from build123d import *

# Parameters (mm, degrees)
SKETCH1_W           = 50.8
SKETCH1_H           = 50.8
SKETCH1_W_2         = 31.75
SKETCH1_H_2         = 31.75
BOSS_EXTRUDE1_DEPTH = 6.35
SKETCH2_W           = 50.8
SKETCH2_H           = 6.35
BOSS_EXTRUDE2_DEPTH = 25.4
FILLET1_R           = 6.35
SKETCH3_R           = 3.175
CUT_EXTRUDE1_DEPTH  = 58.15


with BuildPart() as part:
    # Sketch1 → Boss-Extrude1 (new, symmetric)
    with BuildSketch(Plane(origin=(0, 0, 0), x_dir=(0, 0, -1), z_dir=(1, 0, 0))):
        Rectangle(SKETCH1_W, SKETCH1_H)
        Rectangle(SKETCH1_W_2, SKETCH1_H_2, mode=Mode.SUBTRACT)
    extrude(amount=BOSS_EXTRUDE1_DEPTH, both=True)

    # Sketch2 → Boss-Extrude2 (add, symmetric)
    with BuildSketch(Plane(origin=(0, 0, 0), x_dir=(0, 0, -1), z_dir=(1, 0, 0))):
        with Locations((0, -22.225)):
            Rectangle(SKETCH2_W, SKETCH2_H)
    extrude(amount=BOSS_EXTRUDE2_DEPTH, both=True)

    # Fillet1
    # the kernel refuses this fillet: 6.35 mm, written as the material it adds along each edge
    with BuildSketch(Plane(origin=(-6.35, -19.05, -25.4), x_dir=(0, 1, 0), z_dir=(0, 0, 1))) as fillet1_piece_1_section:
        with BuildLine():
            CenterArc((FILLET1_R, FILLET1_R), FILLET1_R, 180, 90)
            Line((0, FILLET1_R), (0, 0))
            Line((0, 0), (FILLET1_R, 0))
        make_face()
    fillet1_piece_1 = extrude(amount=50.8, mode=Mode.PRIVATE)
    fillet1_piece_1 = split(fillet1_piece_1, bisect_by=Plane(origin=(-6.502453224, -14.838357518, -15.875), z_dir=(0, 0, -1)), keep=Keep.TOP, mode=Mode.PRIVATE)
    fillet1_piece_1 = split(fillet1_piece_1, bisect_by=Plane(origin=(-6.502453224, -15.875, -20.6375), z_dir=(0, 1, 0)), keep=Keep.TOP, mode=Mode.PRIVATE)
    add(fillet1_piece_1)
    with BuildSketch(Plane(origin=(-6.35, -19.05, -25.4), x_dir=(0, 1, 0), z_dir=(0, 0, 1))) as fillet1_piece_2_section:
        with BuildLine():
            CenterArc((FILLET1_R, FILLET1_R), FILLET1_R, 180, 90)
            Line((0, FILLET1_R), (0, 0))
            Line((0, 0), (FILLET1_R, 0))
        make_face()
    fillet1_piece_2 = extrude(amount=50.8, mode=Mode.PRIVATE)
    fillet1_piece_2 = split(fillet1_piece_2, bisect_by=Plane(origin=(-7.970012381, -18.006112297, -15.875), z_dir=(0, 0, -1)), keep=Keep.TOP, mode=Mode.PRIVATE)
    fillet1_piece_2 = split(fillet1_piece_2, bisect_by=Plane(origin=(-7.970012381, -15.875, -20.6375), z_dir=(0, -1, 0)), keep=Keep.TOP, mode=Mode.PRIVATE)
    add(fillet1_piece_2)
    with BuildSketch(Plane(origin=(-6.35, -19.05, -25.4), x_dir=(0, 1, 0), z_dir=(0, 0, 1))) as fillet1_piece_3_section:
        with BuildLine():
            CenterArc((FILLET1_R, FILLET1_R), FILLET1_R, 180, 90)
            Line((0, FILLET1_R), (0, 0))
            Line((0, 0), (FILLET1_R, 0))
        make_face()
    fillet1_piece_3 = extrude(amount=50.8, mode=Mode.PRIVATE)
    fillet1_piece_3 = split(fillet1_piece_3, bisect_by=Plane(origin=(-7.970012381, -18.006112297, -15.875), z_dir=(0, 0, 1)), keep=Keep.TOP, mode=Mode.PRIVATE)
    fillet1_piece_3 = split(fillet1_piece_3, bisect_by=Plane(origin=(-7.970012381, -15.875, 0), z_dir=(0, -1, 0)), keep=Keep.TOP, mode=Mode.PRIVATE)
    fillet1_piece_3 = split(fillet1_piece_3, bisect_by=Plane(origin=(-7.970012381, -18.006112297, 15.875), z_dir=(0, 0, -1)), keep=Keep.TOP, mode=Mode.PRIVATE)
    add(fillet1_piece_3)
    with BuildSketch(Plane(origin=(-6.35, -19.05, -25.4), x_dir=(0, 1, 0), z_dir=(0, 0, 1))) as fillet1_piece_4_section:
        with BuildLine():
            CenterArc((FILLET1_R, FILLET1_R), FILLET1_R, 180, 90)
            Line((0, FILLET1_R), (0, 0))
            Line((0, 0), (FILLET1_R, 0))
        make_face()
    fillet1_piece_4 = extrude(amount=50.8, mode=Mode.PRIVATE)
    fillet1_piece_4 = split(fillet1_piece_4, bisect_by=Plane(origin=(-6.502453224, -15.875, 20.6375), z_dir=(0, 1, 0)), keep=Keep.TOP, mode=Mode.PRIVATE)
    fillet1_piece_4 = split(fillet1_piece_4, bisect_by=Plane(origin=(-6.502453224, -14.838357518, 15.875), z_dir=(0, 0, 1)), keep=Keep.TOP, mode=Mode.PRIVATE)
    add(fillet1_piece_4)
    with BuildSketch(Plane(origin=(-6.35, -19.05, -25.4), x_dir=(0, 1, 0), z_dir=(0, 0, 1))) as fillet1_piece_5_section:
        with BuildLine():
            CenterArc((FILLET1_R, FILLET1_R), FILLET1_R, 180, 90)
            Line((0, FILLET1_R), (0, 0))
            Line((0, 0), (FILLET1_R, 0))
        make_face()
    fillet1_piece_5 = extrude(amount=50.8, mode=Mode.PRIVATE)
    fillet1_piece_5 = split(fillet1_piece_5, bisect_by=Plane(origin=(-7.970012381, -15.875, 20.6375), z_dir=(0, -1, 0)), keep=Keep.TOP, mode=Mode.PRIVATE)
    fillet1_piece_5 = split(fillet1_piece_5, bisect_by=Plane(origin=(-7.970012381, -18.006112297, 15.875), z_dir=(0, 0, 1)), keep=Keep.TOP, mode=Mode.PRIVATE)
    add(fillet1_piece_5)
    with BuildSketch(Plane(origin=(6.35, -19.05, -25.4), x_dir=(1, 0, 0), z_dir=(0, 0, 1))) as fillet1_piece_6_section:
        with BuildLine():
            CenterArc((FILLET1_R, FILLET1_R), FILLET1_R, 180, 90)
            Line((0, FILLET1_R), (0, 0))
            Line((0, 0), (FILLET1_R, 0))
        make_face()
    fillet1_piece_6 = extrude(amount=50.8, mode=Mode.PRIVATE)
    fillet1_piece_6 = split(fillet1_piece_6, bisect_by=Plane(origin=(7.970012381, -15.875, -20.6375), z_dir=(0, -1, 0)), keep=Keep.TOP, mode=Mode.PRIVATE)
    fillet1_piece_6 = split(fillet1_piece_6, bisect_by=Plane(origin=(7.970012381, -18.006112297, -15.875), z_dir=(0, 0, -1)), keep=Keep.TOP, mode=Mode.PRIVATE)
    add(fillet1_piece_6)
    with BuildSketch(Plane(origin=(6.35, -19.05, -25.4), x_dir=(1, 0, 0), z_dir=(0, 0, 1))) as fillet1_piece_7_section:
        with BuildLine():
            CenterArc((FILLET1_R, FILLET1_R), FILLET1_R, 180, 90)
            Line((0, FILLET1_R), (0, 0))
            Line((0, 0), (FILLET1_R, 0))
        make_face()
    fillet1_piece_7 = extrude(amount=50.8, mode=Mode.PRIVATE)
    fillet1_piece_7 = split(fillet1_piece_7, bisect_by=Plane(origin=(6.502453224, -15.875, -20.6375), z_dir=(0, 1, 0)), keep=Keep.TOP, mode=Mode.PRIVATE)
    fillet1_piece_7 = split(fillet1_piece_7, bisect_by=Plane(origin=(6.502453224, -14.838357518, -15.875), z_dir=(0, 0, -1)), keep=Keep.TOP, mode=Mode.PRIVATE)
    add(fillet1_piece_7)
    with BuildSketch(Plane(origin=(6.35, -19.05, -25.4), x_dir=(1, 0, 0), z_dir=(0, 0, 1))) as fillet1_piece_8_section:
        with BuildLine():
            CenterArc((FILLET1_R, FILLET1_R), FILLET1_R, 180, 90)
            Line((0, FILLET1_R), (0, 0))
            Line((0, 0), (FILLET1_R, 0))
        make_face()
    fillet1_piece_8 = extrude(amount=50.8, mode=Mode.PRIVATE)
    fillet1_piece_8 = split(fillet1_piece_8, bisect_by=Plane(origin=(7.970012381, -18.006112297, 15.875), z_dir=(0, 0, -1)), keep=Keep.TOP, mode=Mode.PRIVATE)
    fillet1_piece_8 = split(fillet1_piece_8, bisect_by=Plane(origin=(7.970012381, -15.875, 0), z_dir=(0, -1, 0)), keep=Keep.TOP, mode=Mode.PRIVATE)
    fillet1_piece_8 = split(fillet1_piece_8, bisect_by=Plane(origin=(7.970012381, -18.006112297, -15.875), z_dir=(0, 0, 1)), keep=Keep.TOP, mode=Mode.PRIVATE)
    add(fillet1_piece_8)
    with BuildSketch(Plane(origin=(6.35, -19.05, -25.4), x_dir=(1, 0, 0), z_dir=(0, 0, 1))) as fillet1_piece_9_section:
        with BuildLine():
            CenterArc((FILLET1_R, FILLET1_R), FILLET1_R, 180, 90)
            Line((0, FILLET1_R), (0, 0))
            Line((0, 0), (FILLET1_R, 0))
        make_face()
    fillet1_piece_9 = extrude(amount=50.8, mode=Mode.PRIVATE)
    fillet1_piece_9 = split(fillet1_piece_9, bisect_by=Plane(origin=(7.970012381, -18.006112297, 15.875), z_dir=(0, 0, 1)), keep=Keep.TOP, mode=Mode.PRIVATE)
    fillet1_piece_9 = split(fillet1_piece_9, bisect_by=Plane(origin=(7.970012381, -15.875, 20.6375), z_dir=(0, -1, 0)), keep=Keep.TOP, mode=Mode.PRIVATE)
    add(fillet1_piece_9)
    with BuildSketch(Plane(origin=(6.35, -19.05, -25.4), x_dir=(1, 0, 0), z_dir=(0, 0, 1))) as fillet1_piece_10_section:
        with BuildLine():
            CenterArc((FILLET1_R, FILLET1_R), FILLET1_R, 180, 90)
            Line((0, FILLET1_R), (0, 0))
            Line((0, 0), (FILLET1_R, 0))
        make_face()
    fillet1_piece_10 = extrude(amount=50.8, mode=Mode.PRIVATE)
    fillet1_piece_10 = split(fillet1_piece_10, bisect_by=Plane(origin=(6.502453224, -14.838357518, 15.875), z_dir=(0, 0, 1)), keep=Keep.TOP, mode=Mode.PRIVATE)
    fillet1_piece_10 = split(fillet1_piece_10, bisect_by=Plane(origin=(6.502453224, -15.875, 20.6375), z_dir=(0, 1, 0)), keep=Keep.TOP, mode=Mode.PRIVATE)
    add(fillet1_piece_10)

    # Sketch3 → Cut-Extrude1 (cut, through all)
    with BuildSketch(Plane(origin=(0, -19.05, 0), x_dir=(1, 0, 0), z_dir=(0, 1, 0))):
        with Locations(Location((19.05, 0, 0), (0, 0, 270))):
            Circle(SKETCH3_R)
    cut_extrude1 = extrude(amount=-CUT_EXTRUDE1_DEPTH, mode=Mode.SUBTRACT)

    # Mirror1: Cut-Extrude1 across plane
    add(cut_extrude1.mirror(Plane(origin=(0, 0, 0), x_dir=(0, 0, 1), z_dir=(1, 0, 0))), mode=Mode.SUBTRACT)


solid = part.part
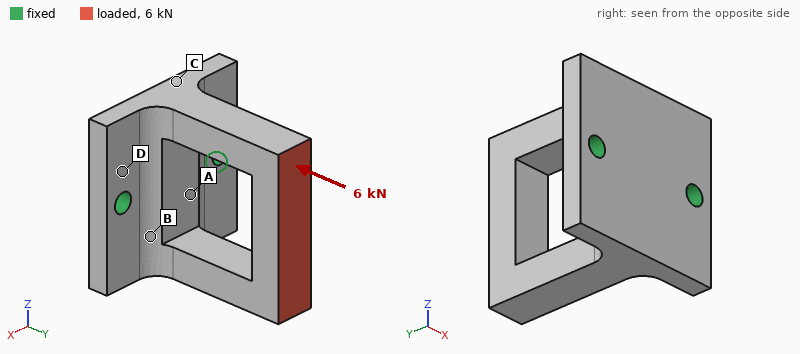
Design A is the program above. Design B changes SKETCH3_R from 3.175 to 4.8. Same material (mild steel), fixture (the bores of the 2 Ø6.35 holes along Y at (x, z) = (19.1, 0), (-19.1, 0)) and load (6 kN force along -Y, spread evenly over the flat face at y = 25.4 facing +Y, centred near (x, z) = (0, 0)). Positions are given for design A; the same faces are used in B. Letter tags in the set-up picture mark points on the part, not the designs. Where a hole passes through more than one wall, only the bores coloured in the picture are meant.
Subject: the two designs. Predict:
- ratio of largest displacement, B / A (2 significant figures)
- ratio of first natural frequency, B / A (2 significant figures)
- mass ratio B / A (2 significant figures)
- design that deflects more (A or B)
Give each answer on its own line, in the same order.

0.90
1.1
0.98
A
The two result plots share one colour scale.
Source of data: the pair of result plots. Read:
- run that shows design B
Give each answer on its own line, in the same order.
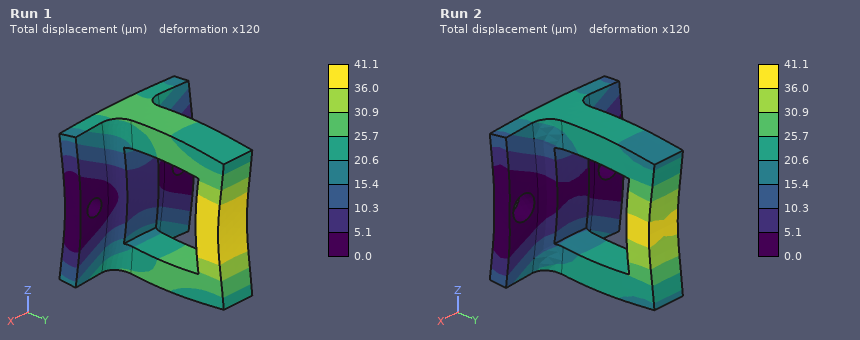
Run 2
